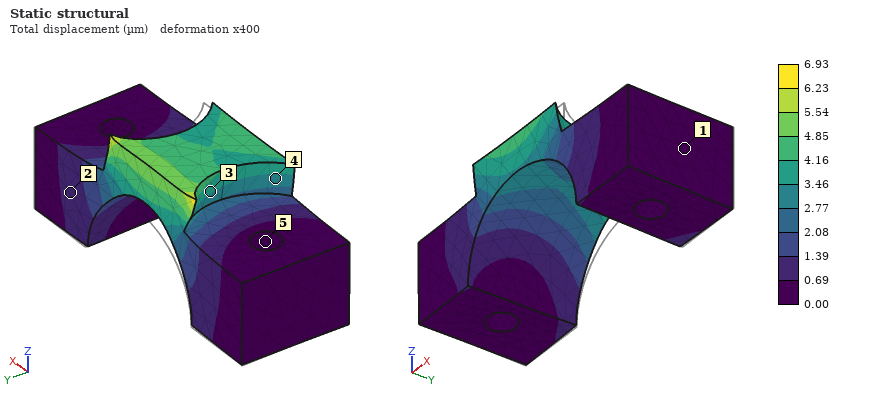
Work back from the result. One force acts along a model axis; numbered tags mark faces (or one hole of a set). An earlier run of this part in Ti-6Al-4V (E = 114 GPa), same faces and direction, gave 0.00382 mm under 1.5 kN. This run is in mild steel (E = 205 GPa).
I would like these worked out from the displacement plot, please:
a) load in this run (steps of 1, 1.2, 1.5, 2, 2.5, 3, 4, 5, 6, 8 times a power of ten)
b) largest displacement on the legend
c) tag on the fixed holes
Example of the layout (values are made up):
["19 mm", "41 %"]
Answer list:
["5 kN", "6.93 µm", "5"]
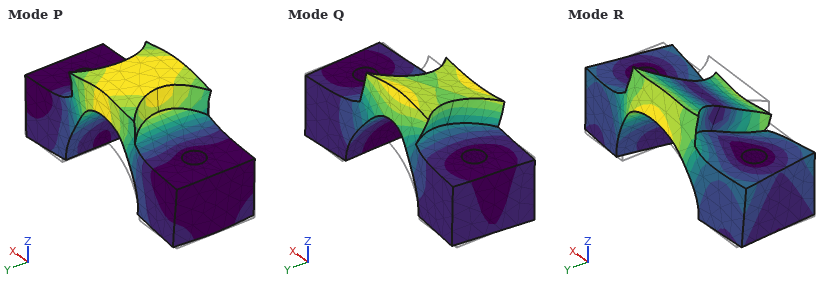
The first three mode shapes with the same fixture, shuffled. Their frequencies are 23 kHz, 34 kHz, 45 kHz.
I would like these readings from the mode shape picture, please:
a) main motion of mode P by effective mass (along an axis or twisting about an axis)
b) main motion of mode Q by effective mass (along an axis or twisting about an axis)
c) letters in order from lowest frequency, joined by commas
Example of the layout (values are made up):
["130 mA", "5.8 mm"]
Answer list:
["along Z", "along Y", "Q, P, R"]
